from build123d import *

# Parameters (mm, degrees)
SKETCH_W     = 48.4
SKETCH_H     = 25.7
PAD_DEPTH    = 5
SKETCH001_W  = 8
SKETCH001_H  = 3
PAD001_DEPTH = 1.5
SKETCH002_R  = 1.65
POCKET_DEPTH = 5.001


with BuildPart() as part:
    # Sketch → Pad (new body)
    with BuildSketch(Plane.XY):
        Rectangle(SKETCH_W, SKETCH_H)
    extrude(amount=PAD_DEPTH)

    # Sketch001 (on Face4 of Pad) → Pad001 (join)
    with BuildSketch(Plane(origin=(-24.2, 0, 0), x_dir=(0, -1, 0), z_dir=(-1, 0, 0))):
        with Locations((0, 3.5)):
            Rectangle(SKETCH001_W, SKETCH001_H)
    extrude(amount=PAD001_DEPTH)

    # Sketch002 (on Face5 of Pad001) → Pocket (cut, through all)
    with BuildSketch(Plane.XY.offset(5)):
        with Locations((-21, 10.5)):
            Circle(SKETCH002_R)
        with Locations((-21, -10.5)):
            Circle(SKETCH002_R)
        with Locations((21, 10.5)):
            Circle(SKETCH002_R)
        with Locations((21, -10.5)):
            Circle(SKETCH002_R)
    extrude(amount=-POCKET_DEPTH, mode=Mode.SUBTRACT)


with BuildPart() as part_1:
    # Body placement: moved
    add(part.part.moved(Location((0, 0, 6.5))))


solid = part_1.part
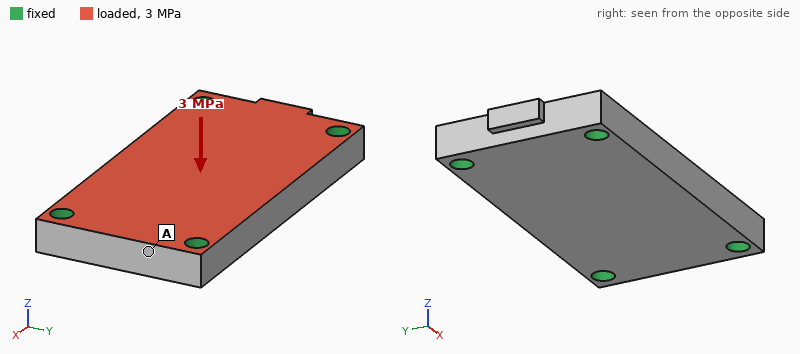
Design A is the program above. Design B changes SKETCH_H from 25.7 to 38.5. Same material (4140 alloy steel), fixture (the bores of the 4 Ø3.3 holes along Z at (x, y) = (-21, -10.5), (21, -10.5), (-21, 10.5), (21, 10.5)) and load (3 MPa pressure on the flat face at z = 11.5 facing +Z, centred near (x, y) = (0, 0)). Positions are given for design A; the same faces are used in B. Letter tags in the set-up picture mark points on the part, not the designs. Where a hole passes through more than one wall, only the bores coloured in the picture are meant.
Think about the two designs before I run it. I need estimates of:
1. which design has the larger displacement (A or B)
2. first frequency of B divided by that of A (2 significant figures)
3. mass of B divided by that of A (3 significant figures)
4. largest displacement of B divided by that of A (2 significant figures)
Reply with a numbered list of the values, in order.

1. B
2. 0.97
3. 1.51
4. 1.1
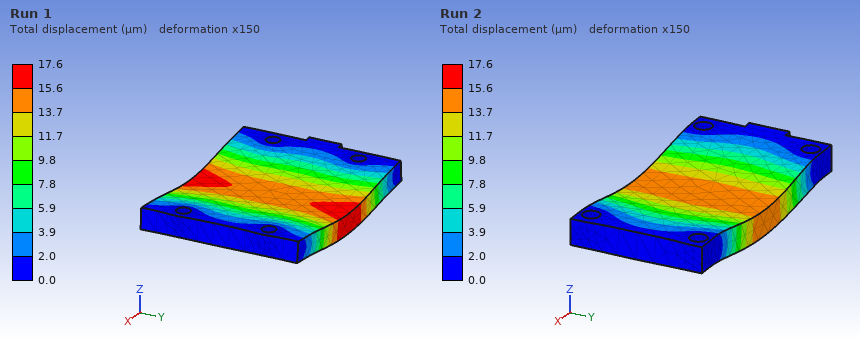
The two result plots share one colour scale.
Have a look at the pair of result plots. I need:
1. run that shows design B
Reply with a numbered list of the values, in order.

1. Run 1
